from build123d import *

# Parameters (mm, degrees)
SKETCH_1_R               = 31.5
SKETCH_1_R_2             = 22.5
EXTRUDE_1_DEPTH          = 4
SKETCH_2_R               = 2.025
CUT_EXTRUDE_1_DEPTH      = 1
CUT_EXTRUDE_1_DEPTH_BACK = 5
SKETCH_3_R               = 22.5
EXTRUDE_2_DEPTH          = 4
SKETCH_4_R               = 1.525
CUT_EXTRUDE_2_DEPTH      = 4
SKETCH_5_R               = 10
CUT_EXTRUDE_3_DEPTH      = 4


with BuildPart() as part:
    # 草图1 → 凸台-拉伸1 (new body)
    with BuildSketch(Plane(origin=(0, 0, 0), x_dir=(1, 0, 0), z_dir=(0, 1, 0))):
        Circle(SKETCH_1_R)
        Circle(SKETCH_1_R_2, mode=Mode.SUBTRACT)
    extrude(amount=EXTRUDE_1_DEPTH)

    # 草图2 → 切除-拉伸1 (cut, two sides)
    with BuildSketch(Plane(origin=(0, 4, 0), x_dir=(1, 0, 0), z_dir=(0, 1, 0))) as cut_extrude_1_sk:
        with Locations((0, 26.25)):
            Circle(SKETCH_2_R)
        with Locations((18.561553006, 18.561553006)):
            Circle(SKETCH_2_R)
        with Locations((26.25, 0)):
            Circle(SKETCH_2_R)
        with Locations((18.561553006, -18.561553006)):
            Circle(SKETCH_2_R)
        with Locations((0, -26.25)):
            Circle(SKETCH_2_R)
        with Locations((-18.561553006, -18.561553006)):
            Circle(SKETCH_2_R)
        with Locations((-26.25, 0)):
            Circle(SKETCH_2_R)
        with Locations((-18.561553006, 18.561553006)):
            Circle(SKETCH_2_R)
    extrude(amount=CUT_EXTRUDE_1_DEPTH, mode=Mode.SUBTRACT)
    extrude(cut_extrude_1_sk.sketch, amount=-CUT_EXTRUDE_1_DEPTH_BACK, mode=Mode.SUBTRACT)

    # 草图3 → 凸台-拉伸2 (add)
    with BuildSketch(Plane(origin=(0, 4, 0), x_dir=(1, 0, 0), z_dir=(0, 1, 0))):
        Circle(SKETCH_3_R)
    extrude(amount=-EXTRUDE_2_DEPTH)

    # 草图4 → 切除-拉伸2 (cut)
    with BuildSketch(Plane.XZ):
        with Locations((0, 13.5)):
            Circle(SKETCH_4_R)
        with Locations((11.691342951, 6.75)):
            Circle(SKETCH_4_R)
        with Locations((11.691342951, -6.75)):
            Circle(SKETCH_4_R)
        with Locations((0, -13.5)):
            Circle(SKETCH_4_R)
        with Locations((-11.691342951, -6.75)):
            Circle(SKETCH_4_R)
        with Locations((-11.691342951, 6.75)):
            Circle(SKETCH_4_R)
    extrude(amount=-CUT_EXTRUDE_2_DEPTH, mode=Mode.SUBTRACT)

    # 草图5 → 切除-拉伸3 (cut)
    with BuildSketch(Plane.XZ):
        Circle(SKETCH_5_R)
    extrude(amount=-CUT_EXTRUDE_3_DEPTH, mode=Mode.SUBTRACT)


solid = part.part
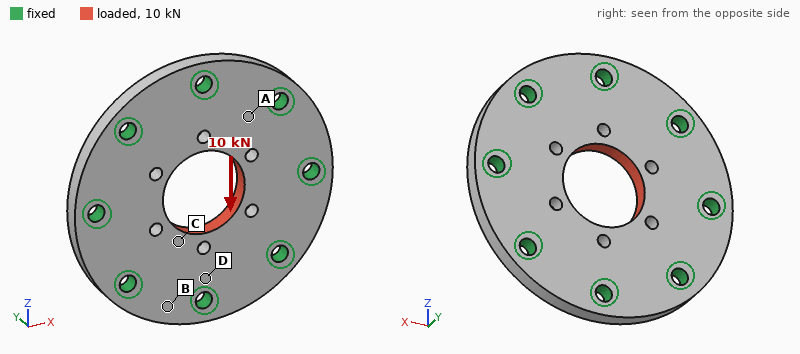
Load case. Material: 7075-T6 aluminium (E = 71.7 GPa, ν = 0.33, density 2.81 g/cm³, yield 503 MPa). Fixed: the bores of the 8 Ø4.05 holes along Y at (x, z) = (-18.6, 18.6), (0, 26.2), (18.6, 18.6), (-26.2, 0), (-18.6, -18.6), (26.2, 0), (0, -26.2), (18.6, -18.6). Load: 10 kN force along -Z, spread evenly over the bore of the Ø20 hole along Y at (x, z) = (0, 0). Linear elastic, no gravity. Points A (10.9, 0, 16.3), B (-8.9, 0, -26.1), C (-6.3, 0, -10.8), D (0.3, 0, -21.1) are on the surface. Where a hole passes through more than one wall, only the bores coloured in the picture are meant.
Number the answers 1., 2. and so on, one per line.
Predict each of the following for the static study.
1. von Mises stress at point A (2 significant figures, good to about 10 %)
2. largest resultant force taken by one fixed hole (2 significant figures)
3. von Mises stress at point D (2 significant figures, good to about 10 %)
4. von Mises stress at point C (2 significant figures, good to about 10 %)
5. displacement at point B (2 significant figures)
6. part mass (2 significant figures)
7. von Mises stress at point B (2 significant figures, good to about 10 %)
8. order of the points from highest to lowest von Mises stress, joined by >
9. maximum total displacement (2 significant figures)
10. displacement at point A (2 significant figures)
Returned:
1. 25 MPa
2. 2.0 kN
3. 52 MPa
4. 36 MPa
5. 3.4 µm
6. 30 g
7. 9.9 MPa
8. D > C > A > B
9. 12 µm
10. 4.2 µm
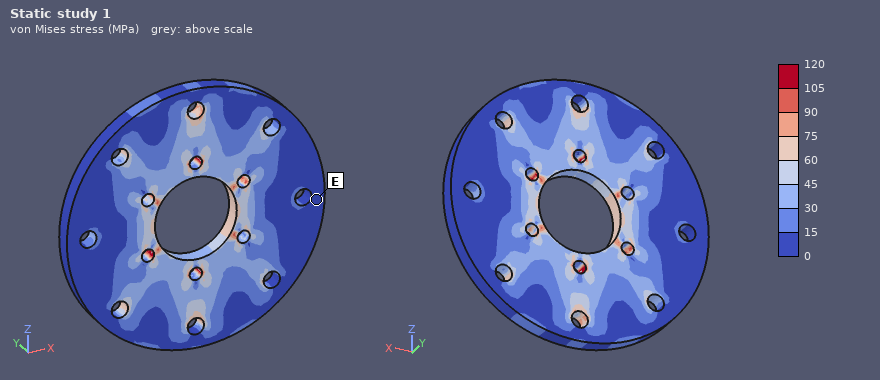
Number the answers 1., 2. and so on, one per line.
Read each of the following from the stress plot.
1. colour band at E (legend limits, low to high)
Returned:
1. 0 to 15 MPa
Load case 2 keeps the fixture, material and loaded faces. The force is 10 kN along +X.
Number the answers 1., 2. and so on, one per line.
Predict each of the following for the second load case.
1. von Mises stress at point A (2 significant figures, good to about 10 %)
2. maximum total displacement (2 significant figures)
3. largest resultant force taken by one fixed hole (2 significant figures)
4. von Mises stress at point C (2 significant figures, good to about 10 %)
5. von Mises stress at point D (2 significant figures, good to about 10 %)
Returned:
1. 27 MPa
2. 12 µm
3. 2.0 kN
4. 46 MPa
5. 14 MPa
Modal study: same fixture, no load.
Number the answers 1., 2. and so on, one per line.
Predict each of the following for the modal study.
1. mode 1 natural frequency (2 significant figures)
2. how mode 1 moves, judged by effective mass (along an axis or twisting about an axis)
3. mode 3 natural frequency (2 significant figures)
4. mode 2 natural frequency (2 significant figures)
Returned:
1. 17 kHz
2. along Y
3. 23 kHz
4. 23 kHz
